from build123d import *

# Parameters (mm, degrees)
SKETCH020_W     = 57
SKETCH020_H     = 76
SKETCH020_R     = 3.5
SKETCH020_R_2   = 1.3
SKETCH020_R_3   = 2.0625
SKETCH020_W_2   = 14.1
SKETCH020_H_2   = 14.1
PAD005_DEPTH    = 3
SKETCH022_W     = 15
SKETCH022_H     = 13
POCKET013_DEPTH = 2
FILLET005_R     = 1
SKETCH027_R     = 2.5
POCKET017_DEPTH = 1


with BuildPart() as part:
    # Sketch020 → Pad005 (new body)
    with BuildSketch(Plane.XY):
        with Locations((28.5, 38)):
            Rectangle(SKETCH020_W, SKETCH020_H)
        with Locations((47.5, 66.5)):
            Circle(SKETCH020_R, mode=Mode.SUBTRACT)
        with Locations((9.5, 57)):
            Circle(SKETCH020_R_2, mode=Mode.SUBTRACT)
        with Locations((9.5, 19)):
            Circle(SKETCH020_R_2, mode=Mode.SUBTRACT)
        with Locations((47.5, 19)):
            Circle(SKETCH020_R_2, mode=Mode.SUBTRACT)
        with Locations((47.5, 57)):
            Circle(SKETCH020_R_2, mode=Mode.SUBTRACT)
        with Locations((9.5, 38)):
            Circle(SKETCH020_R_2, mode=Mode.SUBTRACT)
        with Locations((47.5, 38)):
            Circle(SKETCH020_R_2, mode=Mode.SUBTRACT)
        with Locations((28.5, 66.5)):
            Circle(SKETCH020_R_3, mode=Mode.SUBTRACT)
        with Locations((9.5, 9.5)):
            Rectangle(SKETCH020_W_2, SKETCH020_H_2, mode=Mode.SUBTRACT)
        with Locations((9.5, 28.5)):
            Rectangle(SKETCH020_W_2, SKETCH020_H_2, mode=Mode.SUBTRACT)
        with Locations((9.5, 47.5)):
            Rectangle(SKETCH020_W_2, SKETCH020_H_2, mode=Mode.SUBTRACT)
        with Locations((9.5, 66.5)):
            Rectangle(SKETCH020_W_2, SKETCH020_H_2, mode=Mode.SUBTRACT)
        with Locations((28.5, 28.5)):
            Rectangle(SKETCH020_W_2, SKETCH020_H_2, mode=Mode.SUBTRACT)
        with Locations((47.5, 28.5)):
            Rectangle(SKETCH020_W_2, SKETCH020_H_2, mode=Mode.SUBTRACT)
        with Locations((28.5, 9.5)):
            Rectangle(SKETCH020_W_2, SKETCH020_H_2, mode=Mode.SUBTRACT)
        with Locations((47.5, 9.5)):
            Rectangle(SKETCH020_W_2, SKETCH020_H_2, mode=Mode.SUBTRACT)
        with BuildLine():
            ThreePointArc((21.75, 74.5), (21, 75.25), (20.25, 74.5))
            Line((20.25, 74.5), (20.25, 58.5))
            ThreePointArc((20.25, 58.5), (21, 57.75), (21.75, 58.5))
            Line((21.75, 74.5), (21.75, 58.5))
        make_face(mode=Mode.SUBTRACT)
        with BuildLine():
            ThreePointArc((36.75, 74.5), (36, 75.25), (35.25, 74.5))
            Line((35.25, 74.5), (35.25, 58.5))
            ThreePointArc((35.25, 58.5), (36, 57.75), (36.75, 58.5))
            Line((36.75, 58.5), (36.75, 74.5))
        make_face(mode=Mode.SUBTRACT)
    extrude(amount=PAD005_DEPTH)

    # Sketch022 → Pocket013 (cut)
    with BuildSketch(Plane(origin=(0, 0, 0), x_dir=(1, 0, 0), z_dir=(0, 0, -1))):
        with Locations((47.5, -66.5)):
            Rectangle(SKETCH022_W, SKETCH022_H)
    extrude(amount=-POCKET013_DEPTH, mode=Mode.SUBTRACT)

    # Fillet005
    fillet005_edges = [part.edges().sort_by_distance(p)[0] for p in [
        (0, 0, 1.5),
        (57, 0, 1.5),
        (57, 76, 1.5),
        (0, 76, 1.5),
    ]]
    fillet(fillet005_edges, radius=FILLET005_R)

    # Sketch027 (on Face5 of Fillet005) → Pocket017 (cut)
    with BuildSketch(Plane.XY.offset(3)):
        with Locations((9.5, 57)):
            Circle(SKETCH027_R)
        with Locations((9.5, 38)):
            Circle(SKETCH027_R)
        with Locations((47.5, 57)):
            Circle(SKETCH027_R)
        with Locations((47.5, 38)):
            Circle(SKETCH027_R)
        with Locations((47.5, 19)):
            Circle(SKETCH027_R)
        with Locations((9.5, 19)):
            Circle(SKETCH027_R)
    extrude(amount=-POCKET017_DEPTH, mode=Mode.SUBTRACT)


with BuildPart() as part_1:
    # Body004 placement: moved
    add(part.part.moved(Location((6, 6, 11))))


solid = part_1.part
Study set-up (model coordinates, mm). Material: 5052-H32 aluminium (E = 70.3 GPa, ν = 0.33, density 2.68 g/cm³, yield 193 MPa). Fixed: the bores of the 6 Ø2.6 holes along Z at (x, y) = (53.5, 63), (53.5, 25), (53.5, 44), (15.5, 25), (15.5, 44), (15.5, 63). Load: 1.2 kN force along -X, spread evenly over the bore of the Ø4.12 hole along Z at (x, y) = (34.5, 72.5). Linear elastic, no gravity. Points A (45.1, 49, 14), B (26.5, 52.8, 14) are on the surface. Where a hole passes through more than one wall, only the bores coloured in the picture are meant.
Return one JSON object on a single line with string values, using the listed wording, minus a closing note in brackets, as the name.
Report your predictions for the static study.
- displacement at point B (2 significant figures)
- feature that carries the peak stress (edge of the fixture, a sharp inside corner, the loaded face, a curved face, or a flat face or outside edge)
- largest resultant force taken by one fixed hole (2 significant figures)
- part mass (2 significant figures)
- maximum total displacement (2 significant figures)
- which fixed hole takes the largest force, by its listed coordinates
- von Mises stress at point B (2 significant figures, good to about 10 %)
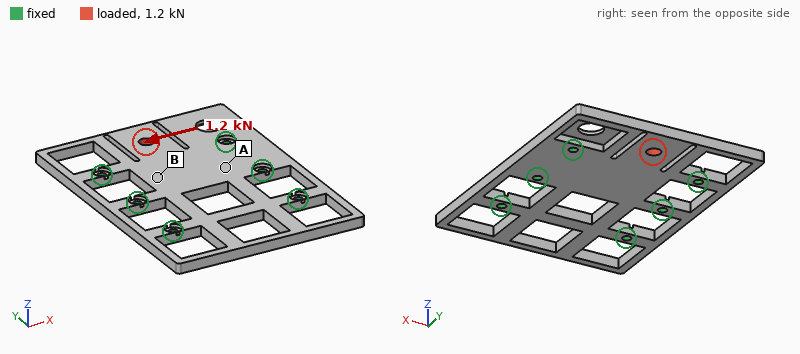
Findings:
{"displacement at point B": "6.9 µm", "feature that carries the peak stress": "a curved face", "largest resultant force taken by one fixed hole": "780 N", "part mass": "20 g", "maximum total displacement": "37 µm", "which fixed hole takes the largest force, by its listed coordinates": "(53.5, 63)", "von Mises stress at point B": "16 MPa"}
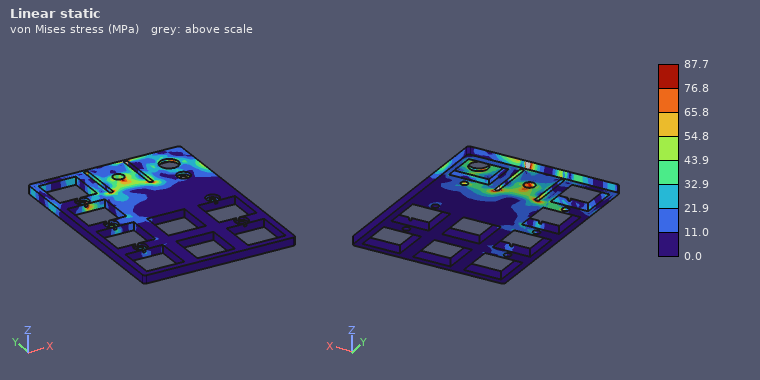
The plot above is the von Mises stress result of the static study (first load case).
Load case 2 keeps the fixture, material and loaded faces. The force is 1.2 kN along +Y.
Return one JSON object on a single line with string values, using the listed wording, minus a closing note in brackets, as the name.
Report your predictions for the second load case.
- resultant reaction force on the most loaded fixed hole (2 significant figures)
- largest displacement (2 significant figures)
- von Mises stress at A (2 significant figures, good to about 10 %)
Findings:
{"resultant reaction force on the most loaded fixed hole": "520 N", "largest displacement": "18 µm", "von Mises stress at A": "17 MPa"}
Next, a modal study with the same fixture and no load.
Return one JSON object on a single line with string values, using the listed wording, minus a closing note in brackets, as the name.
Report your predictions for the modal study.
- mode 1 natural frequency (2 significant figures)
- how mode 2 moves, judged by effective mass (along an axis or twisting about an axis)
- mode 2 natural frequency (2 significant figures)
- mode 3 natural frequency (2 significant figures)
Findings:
{"mode 1 natural frequency": "3400 Hz", "how mode 2 moves, judged by effective mass": "along Z", "mode 2 natural frequency": "3500 Hz", "mode 3 natural frequency": "4700 Hz"}
